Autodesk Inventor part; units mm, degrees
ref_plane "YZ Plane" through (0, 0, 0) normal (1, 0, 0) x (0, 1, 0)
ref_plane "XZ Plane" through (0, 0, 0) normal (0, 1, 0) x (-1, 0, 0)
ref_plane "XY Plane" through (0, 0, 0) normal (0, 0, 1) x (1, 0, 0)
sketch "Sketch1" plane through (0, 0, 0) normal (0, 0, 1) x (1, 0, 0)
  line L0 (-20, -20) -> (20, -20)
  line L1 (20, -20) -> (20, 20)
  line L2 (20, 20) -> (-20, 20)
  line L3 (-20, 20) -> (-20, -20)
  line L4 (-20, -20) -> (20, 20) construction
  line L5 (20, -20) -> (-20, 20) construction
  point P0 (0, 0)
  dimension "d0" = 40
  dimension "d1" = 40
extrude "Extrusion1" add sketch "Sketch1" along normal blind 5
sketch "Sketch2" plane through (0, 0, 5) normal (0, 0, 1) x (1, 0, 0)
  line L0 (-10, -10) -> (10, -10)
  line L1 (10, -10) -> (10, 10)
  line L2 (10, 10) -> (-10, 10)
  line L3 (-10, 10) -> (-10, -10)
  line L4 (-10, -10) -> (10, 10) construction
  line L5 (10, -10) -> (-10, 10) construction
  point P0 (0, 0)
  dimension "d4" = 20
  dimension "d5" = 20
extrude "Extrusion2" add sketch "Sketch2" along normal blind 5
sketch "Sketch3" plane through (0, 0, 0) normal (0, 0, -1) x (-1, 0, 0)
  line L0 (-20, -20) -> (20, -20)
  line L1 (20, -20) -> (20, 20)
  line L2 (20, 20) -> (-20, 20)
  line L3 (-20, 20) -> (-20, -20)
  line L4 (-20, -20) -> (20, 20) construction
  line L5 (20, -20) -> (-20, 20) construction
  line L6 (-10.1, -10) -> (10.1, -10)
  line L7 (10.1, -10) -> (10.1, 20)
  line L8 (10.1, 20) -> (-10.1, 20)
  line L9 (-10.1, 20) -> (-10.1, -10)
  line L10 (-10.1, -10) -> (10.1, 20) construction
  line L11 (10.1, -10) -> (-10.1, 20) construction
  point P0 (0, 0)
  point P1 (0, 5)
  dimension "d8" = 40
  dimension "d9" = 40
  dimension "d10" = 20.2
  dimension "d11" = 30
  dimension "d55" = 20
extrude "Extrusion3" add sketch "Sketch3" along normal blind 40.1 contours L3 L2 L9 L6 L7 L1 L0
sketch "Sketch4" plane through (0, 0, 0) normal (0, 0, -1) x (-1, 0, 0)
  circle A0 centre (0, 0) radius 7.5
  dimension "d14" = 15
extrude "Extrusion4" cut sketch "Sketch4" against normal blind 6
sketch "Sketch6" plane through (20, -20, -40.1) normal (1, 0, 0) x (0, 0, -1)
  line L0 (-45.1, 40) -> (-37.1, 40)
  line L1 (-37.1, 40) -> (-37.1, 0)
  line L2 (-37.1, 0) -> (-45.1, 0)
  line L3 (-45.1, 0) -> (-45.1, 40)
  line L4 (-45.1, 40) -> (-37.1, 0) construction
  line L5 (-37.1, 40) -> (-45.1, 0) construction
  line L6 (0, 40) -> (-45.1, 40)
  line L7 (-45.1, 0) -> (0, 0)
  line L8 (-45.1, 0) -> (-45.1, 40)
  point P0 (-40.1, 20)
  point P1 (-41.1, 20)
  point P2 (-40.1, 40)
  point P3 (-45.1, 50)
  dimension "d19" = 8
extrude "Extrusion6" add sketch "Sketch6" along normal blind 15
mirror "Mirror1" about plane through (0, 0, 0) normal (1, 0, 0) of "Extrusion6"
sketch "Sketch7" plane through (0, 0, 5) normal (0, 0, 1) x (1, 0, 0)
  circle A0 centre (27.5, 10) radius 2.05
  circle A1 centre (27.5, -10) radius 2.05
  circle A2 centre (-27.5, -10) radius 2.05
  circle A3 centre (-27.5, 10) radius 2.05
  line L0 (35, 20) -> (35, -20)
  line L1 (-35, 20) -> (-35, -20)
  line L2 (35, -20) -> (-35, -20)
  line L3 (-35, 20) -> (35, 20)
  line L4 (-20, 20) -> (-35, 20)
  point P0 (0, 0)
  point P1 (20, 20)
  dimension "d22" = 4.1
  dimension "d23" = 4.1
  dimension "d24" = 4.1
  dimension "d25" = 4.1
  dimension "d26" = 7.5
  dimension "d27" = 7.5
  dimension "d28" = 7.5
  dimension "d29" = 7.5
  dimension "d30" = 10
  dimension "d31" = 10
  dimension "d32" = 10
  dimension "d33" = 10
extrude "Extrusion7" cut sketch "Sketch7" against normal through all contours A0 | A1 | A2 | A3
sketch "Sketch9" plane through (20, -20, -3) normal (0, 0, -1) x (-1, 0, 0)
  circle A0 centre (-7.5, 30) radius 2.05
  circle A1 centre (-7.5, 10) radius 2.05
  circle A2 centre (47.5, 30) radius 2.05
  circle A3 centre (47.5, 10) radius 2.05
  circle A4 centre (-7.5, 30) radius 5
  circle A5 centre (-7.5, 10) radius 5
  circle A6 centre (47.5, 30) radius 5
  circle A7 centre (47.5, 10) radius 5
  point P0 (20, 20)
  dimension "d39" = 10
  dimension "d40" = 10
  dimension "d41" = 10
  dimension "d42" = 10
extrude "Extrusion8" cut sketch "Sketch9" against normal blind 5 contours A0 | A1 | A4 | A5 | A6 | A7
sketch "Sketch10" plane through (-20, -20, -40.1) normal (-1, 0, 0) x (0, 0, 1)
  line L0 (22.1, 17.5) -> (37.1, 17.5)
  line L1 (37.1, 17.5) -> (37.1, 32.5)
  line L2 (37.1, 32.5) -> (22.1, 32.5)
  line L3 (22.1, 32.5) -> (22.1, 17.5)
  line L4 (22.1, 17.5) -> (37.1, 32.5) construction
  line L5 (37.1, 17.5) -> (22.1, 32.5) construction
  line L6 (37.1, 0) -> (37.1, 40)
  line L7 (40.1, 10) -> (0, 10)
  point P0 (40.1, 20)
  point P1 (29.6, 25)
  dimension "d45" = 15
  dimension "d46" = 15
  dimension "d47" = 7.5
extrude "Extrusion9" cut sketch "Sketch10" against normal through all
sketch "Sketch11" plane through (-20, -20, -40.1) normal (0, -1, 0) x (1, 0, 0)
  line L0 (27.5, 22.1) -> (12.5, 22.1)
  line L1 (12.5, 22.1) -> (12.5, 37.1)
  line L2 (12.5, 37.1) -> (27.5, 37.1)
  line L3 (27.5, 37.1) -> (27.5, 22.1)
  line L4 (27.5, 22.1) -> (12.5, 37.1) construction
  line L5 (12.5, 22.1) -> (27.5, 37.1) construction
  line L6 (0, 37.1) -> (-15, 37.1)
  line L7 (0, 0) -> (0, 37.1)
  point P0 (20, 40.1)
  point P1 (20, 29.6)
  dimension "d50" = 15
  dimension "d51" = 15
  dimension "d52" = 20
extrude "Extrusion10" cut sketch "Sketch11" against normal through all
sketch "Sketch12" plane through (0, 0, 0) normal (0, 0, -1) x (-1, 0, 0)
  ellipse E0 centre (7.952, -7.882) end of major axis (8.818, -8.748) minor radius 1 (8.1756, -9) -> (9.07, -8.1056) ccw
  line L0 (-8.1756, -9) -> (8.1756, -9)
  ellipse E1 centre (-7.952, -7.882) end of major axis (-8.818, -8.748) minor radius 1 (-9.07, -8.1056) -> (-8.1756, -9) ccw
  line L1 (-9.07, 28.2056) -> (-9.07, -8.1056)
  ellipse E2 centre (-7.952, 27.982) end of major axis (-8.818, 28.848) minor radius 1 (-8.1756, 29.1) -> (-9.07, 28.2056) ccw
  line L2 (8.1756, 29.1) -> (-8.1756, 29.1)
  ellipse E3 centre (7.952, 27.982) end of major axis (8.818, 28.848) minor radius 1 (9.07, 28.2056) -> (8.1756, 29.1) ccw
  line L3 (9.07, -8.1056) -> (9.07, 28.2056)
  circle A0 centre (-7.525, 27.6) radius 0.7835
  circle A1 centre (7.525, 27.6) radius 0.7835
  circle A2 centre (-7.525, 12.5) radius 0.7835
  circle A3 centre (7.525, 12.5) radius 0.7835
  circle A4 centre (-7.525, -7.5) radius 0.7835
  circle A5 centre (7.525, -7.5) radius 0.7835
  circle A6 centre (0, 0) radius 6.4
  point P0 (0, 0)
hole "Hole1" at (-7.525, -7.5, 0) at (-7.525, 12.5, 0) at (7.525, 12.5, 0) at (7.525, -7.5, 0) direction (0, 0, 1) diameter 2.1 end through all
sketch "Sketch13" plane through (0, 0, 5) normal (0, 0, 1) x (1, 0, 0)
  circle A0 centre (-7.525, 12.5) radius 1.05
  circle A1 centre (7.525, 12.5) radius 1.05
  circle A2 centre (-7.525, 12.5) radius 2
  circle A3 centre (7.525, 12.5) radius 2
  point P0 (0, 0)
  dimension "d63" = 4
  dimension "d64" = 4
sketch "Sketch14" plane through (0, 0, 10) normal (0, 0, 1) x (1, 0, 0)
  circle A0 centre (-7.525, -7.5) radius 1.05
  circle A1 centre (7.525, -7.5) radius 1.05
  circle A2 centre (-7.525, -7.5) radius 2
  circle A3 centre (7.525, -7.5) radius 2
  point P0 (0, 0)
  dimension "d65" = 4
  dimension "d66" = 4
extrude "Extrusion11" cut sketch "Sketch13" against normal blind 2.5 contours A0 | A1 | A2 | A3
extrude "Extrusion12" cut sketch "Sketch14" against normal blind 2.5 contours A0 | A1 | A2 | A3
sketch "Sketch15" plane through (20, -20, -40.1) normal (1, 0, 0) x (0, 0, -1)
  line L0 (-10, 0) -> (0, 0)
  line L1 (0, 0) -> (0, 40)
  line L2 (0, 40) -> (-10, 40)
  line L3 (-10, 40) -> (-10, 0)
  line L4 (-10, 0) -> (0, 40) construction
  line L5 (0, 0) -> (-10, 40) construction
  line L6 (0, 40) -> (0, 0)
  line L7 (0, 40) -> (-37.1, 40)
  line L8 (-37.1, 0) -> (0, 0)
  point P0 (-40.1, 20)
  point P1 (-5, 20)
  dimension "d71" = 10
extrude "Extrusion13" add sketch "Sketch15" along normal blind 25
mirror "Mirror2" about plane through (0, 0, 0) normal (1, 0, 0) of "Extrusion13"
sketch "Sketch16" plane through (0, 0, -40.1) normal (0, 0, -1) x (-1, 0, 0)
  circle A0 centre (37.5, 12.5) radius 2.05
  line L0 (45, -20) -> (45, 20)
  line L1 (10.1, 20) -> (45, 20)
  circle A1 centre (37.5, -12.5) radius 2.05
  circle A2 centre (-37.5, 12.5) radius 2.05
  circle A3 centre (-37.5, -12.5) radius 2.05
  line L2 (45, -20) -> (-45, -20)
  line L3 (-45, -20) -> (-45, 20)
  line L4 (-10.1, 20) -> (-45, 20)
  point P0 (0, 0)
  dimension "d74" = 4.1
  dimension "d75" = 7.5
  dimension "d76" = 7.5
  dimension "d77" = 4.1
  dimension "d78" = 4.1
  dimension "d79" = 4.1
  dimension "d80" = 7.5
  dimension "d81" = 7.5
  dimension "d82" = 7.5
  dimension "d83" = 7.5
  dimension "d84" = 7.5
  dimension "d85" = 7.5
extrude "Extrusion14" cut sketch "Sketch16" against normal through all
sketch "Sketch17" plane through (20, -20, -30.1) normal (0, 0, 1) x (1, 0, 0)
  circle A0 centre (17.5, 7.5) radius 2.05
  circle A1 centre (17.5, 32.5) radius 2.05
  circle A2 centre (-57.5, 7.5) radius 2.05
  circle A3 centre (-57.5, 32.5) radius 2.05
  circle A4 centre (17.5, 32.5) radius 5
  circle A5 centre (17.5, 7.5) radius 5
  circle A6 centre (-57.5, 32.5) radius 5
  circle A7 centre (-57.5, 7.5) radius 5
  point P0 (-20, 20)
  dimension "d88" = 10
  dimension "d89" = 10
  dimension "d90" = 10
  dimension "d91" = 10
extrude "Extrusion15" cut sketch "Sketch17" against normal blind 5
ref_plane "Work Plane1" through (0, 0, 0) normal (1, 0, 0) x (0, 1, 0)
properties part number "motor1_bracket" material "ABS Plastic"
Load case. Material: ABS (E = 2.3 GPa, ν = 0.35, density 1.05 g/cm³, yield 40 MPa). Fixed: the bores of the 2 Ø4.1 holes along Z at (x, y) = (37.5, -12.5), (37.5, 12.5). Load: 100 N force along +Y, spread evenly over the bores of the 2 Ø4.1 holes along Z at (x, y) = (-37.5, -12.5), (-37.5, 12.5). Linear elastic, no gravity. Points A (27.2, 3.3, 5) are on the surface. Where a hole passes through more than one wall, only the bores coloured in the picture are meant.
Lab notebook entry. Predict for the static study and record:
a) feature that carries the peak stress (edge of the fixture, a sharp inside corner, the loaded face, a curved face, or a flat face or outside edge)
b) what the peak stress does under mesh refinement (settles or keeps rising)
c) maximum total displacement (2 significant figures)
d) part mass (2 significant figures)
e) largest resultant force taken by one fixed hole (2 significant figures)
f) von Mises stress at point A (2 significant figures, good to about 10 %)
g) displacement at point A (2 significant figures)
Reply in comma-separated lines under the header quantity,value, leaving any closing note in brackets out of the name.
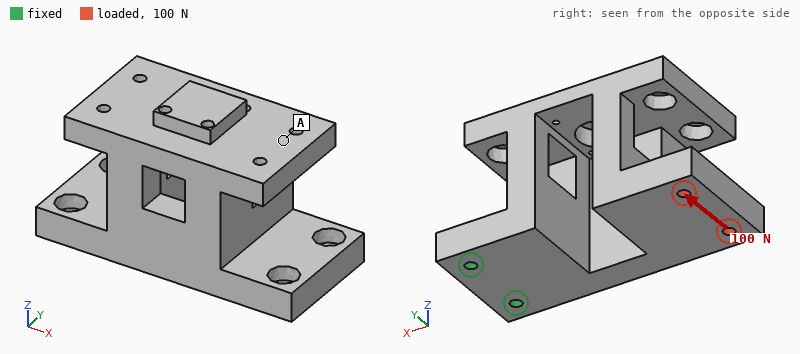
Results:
quantity,value
feature that carries the peak stress,edge of the fixture
what the peak stress does under mesh refinement,keeps rising
maximum total displacement,1.2 mm
part mass,71 g
largest resultant force taken by one fixed hole,290 N
von Mises stress at point A,1.1 MPa
displacement at point A,0.21 mm
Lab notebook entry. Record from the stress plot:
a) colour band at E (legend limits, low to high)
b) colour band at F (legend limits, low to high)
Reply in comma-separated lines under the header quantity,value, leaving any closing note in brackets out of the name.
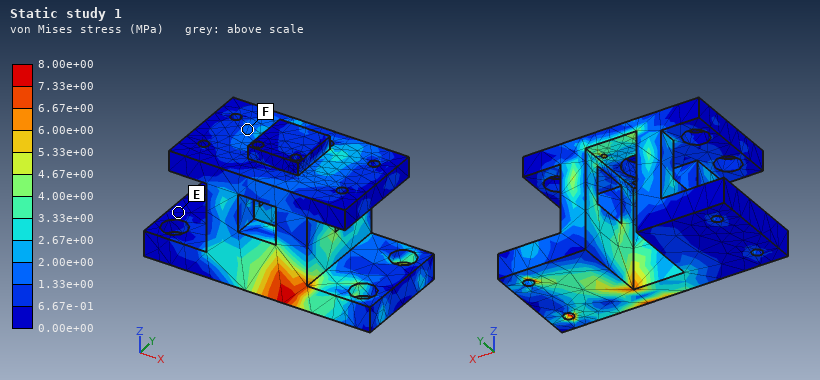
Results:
quantity,value
colour band at E,0.00e+00 to 6.67e-01 MPa
colour band at F,1.33e+00 to 2.00e+00 MPa
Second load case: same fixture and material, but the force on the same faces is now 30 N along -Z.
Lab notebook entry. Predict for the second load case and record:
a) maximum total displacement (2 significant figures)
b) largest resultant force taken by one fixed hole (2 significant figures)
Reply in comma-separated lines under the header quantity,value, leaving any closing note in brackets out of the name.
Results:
quantity,value
maximum total displacement,1.0 mm
largest resultant force taken by one fixed hole,16 N
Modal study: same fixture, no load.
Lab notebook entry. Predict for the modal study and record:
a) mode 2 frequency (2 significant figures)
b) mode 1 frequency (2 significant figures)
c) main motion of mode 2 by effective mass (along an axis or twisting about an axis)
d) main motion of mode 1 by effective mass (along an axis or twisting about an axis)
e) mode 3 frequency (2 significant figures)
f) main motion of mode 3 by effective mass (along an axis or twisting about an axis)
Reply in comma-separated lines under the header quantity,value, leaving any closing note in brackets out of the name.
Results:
quantity,value
mode 2 frequency,420 Hz
mode 1 frequency,170 Hz
main motion of mode 2 by effective mass,along Y
main motion of mode 1 by effective mass,along Z
mode 3 frequency,600 Hz
main motion of mode 3 by effective mass,along Y
